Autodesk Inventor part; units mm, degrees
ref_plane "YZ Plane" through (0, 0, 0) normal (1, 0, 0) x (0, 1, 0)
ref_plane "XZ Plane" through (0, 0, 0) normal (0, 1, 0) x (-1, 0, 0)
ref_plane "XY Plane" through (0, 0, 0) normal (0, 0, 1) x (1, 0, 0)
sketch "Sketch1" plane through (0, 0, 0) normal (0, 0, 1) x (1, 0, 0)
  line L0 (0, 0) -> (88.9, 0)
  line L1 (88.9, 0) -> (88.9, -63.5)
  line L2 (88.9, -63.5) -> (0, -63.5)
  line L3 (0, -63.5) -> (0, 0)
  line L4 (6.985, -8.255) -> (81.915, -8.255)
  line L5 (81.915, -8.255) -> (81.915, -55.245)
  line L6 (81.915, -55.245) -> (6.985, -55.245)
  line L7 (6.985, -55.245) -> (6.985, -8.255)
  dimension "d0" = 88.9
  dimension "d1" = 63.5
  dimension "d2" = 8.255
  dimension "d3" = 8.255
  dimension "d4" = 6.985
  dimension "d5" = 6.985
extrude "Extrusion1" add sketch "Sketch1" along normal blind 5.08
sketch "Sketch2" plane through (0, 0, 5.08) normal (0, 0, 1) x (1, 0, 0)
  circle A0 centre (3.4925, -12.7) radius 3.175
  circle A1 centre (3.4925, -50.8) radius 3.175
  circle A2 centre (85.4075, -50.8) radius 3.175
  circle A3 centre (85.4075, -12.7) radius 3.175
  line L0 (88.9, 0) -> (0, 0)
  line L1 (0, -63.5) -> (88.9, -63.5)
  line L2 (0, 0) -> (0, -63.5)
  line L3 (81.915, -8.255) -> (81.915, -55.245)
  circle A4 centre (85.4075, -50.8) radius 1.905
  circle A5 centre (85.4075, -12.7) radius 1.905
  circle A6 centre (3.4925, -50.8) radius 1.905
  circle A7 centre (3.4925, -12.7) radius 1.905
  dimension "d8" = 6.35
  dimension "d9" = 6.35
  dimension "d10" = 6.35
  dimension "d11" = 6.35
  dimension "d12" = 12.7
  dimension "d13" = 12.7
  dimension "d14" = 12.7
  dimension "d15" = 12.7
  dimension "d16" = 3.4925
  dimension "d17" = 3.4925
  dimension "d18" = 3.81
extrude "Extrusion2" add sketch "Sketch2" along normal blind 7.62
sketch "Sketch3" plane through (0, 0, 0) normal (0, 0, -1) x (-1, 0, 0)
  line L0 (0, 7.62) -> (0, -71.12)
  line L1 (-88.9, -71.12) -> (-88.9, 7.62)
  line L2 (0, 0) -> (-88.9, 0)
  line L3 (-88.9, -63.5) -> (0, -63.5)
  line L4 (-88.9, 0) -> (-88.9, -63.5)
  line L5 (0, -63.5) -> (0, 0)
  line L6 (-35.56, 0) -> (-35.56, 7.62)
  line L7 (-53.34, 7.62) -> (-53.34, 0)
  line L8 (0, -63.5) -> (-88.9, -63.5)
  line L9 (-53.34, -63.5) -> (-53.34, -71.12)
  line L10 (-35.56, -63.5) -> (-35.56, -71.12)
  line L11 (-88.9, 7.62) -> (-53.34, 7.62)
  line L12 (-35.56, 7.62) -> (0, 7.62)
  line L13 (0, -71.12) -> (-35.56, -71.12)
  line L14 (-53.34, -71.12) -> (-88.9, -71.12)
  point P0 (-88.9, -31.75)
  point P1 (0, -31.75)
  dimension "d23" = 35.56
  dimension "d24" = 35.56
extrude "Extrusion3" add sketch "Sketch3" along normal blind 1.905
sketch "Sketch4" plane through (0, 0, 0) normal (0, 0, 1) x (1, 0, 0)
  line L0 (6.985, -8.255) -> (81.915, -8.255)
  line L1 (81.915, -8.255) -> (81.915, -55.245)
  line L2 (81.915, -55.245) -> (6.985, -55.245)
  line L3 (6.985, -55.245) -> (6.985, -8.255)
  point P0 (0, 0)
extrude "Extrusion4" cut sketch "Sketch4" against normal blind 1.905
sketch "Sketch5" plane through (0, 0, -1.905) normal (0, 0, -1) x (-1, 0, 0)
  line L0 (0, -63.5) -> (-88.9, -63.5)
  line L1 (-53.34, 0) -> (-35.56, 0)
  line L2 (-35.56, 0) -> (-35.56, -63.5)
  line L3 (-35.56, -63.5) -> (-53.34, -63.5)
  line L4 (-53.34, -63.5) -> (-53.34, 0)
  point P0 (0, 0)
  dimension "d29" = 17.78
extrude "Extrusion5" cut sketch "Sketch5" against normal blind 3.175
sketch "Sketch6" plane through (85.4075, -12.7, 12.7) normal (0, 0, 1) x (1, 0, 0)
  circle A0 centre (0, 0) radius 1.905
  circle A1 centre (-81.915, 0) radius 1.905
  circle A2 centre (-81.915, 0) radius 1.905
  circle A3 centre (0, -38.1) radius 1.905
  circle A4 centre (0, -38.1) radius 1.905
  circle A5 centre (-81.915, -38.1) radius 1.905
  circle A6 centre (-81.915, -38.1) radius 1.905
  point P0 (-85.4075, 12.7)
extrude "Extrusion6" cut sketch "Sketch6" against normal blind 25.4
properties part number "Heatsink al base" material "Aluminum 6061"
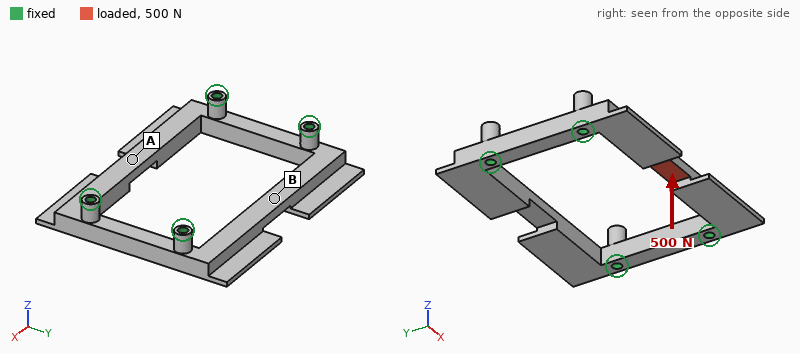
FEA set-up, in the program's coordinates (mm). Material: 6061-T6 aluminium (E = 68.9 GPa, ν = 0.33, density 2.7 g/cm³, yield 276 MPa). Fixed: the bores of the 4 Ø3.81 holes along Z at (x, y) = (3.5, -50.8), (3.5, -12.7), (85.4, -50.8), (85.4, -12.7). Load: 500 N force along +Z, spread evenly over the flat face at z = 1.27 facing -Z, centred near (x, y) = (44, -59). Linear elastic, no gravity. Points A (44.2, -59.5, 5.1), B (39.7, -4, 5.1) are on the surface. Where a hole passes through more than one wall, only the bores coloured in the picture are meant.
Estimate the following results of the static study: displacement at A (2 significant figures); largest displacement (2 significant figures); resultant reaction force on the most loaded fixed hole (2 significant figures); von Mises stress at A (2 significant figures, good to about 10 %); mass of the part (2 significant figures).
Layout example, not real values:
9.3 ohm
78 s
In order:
0.23 mm
0.24 mm
460 N
130 MPa
44 g
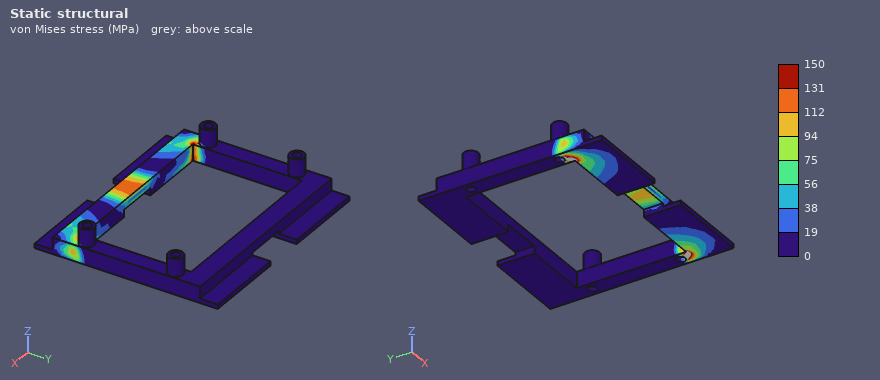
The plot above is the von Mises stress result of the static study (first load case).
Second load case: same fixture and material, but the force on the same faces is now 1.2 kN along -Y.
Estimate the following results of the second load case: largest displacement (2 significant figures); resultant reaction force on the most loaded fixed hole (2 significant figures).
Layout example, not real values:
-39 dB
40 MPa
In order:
0.25 mm
1.2 kN
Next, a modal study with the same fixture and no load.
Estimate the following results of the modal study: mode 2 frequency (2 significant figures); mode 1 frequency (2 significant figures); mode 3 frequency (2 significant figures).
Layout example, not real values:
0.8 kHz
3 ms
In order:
3400 Hz
3400 Hz
5100 Hz
